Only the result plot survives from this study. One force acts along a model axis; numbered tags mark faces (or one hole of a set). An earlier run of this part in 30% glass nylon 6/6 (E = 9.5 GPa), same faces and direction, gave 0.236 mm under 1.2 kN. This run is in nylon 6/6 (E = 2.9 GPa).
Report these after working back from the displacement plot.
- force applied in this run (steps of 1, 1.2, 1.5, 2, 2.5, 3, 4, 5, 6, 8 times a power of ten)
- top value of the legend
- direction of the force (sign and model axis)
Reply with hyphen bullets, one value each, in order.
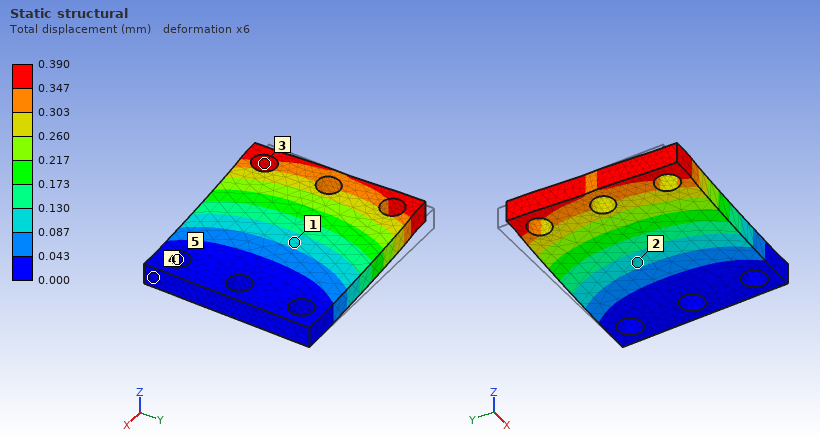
- 600 N
- 0.390 mm
- -Y
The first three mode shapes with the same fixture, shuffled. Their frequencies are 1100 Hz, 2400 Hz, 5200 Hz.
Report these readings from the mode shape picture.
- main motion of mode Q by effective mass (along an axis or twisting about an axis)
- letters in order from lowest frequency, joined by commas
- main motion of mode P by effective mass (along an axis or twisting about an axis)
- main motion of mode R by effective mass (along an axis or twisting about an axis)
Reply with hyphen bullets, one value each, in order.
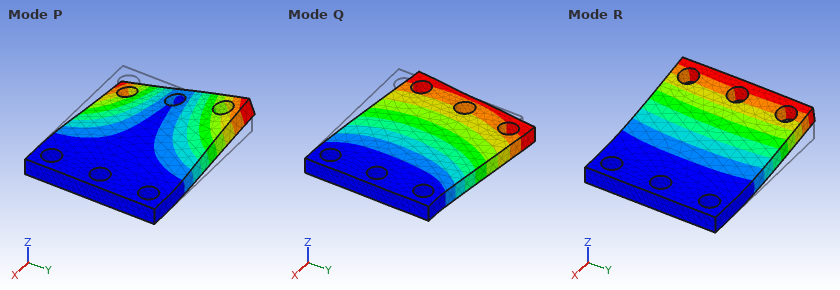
- along Y
- R, P, Q
- twisting about X
- along Z
